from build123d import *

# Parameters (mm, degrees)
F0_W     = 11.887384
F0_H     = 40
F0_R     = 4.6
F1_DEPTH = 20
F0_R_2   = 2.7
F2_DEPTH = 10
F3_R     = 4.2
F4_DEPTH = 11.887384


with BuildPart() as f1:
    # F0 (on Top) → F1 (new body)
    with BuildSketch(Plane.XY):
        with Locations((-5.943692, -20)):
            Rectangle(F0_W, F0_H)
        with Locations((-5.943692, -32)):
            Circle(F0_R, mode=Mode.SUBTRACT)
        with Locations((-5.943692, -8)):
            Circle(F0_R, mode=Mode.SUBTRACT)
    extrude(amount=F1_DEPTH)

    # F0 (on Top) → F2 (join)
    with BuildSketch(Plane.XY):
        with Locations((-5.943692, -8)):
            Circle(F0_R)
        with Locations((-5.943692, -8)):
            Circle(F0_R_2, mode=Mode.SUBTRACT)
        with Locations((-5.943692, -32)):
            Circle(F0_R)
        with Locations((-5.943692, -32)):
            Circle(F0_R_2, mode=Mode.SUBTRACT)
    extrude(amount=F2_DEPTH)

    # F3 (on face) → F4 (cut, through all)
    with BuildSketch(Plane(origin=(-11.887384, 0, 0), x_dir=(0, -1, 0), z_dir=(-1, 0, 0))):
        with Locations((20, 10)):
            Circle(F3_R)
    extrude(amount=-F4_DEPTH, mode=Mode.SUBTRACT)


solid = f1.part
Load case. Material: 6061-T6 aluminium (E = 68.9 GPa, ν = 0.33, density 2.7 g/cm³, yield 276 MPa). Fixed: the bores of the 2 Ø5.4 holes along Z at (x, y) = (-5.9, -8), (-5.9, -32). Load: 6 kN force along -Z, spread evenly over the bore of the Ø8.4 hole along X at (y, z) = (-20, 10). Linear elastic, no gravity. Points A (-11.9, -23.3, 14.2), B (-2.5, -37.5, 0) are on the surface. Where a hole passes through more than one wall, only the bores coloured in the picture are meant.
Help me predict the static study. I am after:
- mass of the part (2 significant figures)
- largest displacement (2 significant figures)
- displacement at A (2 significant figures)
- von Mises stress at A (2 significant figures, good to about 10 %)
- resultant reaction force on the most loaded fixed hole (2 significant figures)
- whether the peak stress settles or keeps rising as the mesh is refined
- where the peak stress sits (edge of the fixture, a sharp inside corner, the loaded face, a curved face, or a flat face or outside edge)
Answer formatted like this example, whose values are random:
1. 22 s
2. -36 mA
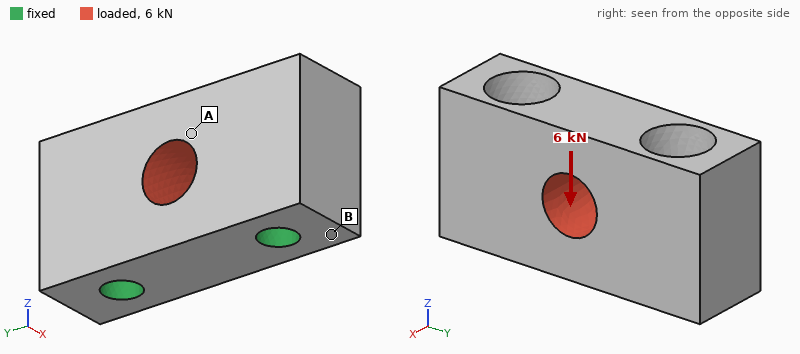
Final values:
1. 19 g
2. 9.0 µm
3. 7.5 µm
4. 27 MPa
5. 3.1 kN
6. keeps rising
7. edge of the fixture
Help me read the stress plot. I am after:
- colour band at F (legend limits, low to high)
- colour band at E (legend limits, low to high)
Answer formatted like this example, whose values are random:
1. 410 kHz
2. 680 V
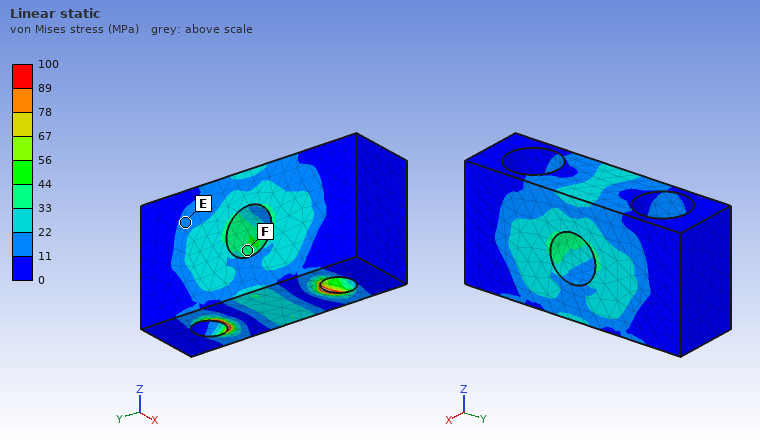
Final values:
1. 33 to 44 MPa
2. 11 to 22 MPa
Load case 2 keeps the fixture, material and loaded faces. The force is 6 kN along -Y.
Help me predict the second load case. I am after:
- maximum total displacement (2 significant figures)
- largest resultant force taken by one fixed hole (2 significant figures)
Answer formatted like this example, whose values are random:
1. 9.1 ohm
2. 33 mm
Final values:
1. 8.7 µm
2. 3.1 kN
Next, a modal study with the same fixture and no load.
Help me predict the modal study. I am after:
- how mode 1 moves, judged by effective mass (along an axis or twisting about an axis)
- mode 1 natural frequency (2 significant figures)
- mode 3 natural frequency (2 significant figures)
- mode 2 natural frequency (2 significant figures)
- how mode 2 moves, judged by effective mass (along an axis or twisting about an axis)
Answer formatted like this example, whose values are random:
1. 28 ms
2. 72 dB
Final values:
1. along X
2. 25 kHz
3. 36 kHz
4. 33 kHz
5. twisting about Z
